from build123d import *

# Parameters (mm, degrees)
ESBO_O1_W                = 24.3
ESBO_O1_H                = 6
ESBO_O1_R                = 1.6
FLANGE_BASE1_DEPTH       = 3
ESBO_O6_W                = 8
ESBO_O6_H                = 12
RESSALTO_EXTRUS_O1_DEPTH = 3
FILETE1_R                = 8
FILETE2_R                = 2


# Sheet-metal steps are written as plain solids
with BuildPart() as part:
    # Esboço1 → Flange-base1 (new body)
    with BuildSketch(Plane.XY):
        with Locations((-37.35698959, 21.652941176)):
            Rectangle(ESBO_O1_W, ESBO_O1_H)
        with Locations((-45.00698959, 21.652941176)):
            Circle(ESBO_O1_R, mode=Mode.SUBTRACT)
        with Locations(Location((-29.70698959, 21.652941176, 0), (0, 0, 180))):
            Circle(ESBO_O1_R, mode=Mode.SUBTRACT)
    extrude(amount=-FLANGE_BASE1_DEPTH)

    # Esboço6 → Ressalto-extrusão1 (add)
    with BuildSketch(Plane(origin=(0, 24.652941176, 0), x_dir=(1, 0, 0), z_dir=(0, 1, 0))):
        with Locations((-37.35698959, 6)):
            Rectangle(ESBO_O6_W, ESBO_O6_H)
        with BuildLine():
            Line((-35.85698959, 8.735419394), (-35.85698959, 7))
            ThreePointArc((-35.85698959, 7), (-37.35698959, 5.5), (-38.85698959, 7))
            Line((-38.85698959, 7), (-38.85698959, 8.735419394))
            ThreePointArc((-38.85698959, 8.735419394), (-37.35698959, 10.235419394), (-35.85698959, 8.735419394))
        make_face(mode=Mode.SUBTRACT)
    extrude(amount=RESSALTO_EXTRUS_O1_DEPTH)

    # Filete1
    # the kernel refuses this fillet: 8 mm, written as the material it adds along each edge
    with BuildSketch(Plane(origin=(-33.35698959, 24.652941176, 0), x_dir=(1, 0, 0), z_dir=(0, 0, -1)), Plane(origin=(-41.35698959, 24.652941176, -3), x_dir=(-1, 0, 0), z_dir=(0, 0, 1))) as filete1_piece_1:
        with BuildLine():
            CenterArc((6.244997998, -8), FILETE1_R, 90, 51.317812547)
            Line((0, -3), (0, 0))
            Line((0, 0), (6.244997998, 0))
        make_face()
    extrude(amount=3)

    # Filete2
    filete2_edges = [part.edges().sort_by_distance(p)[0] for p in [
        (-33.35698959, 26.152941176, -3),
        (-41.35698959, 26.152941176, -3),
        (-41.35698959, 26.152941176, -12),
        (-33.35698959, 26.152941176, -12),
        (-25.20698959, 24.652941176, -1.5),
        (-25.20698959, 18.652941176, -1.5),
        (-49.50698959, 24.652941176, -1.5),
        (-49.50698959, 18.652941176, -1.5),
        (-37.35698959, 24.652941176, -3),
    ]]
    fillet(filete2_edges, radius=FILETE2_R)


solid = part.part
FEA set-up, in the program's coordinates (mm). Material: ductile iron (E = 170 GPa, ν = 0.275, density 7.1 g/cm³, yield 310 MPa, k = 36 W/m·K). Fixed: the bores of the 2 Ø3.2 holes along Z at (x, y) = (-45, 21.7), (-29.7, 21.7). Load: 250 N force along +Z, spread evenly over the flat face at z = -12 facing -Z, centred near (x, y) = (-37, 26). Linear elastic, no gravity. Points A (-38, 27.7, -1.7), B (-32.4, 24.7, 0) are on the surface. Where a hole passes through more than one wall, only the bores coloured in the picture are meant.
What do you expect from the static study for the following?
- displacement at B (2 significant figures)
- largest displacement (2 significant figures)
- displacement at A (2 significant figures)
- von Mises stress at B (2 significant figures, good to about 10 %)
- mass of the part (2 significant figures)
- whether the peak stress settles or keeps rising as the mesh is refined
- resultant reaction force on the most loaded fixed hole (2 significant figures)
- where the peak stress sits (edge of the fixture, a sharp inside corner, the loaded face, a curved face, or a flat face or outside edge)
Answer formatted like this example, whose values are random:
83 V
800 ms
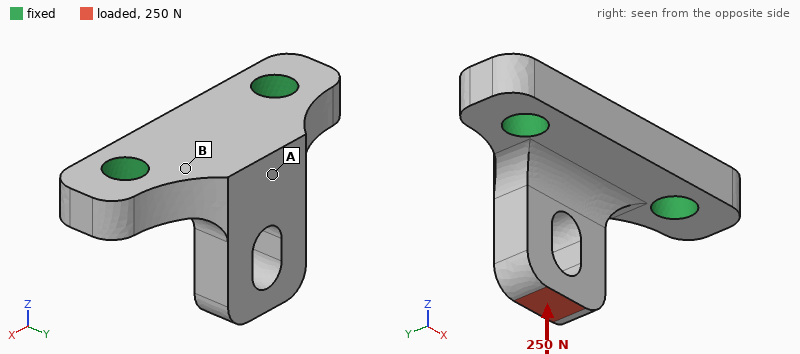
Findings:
1.4 µm
8.2 µm
3.5 µm
27 MPa
4.8 g
keeps rising
130 N
edge of the fixture
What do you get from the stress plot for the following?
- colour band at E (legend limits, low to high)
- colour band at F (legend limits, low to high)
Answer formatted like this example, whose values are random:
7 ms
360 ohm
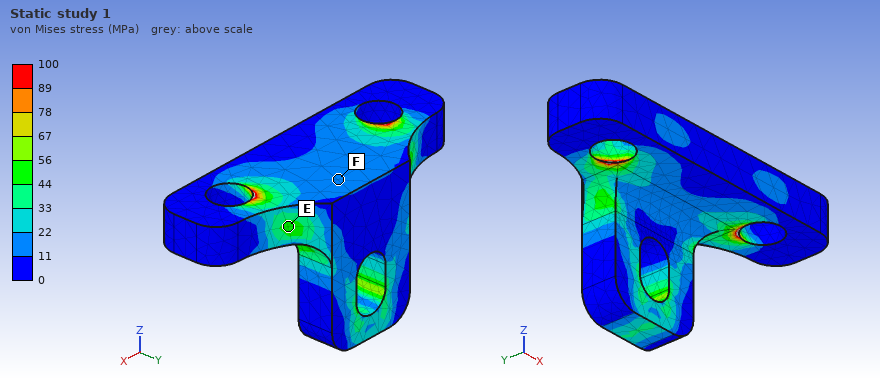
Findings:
44 to 56 MPa
11 to 22 MPa
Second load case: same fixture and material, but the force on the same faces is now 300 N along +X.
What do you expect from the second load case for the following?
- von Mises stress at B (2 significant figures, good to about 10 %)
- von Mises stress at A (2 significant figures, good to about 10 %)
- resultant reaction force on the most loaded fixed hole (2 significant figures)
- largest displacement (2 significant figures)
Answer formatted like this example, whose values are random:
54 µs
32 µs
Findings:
32 MPa
45 MPa
310 N
15 µm
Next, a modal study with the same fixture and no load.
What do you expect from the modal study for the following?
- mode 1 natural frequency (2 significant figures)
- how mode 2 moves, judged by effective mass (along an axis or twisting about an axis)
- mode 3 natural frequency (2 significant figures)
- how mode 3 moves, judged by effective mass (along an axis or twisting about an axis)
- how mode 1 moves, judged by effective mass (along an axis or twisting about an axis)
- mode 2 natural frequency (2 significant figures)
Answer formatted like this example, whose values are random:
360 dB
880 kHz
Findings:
18 kHz
along X
43 kHz
along Z
along Y
34 kHz
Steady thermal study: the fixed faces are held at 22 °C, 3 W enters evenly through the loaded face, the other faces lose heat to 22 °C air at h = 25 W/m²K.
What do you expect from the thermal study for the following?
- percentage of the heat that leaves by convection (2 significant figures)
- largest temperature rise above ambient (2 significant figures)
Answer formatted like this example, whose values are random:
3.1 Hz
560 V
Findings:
6.9 %
59 K
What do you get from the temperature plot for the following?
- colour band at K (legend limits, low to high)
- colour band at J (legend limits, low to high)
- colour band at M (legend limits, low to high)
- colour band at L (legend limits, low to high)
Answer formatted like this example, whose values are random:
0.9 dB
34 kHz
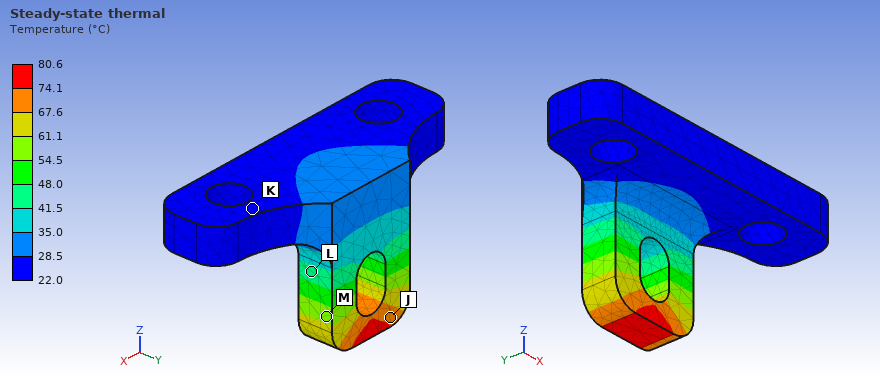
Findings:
22.0 to 28.5 °C
67.6 to 74.1 °C
54.5 to 61.1 °C
41.5 to 48.0 °C
